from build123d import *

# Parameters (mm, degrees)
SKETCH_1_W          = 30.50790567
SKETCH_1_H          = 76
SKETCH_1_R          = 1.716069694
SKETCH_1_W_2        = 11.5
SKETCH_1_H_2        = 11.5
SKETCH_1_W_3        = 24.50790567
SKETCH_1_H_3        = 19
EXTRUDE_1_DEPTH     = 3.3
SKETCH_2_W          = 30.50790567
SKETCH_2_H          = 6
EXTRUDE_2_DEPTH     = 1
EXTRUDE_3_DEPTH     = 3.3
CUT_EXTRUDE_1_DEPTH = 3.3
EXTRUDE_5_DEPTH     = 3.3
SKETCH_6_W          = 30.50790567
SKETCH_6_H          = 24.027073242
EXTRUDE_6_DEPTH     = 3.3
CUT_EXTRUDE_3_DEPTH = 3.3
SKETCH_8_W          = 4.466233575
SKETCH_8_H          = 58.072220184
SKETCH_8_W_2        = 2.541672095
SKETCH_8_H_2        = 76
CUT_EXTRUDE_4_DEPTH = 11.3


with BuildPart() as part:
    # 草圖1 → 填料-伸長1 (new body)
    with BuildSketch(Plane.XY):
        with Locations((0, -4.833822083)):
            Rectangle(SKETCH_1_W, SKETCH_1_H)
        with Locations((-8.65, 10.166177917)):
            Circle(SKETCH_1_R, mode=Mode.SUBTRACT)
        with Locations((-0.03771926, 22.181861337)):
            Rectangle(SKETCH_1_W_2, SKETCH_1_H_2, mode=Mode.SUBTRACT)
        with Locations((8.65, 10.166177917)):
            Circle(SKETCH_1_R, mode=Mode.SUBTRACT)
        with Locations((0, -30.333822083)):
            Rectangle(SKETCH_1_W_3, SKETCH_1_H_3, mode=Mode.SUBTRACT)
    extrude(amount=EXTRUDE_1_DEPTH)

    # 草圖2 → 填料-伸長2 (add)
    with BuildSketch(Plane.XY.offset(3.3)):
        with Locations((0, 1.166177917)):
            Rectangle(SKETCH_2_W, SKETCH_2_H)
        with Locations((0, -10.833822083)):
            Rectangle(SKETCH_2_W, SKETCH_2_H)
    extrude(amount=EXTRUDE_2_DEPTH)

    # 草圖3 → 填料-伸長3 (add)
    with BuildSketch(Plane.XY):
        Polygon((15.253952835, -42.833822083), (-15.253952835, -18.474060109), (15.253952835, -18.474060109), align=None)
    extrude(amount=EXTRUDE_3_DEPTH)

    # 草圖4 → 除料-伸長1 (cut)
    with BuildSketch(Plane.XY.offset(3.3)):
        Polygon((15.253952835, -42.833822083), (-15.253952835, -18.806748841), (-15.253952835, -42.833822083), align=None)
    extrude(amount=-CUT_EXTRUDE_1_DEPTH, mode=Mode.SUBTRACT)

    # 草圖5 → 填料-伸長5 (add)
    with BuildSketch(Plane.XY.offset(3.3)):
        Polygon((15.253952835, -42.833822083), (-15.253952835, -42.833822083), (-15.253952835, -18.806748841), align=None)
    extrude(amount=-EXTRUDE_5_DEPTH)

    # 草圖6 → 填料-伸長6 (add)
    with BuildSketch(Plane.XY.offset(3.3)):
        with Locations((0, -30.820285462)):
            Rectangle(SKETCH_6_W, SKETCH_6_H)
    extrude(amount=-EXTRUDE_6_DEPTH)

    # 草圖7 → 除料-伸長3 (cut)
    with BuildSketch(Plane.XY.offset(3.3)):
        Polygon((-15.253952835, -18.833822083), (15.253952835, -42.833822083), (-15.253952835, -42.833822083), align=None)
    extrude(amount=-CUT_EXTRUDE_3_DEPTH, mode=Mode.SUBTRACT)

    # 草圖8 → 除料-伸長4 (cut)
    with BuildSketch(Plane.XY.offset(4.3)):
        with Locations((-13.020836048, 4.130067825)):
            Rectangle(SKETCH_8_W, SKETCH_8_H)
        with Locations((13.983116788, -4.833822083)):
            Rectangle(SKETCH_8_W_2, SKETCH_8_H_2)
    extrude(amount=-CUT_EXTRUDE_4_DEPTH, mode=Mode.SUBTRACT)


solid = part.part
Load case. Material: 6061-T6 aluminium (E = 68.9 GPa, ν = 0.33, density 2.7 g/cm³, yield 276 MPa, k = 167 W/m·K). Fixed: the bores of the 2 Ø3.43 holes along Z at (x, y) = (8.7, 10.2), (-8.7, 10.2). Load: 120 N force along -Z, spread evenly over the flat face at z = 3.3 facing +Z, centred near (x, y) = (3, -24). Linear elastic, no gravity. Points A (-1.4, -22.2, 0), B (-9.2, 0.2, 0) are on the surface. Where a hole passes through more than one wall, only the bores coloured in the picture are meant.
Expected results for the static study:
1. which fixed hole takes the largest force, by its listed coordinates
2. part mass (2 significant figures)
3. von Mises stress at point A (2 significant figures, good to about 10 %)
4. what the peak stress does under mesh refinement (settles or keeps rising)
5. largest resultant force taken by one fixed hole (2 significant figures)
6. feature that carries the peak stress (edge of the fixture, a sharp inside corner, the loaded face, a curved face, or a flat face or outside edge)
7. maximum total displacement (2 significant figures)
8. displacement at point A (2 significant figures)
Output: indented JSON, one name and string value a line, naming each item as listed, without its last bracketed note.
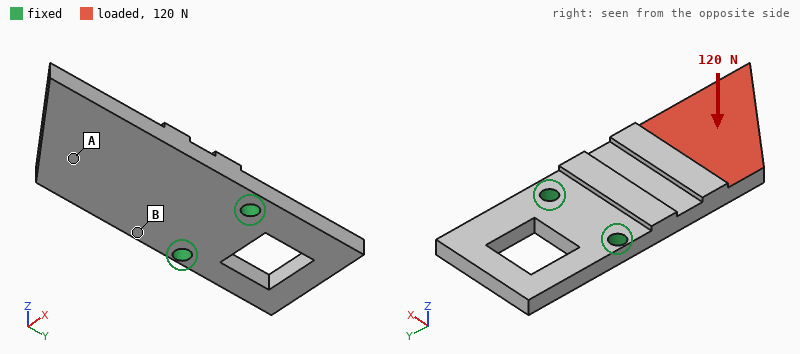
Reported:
{
  "which fixed hole takes the largest force, by its listed coordinates": "(8.7, 10.2)",
  "part mass": "13 g",
  "von Mises stress at point A": "12 MPa",
  "what the peak stress does under mesh refinement": "keeps rising",
  "largest resultant force taken by one fixed hole": "84 N",
  "feature that carries the peak stress": "edge of the fixture",
  "maximum total displacement": "0.48 mm",
  "displacement at point A": "0.24 mm"
}
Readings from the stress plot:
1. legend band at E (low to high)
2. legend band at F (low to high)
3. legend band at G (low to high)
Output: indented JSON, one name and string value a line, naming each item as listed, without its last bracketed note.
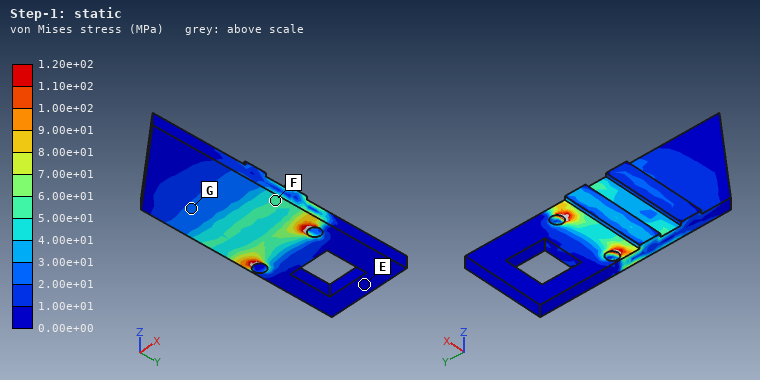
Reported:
{
  "legend band at E": "0.00e+00 to 1.00e+01 MPa",
  "legend band at F": "5.00e+01 to 6.00e+01 MPa",
  "legend band at G": "2.00e+01 to 3.00e+01 MPa"
}
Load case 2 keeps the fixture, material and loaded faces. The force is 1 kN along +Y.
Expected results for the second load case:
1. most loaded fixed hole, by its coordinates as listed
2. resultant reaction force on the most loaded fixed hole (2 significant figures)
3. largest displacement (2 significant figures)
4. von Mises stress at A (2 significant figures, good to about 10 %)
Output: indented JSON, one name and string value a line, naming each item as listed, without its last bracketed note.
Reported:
{
  "most loaded fixed hole, by its coordinates as listed": "(8.7, 10.2)",
  "resultant reaction force on the most loaded fixed hole": "660 N",
  "largest displacement": "0.31 mm",
  "von Mises stress at A": "16 MPa"
}
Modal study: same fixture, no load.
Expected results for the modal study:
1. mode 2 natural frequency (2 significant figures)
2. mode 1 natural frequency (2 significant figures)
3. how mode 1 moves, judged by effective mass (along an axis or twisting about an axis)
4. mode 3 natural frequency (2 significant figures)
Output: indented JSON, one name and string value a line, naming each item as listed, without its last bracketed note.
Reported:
{
  "mode 2 natural frequency": "4700 Hz",
  "mode 1 natural frequency": "1600 Hz",
  "how mode 1 moves, judged by effective mass": "along Z",
  "mode 3 natural frequency": "6400 Hz"
}
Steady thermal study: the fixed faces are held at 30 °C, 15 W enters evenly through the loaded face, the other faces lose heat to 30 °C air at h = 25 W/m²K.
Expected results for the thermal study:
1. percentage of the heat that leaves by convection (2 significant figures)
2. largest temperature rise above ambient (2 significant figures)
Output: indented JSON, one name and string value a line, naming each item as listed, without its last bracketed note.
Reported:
{
  "percentage of the heat that leaves by convection": "6.6 %",
  "largest temperature rise above ambient": "39 K"
}
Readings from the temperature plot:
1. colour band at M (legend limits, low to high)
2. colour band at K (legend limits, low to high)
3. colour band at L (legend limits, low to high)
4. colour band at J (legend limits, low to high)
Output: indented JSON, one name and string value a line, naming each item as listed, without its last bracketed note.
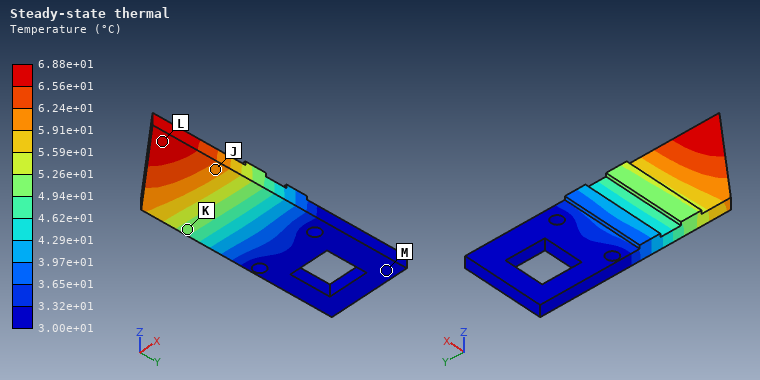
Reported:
{
  "colour band at M": "3.00e+01 to 3.32e+01 °C",
  "colour band at K": "4.94e+01 to 5.26e+01 °C",
  "colour band at L": "6.56e+01 to 6.88e+01 °C",
  "colour band at J": "5.91e+01 to 6.24e+01 °C"
}
